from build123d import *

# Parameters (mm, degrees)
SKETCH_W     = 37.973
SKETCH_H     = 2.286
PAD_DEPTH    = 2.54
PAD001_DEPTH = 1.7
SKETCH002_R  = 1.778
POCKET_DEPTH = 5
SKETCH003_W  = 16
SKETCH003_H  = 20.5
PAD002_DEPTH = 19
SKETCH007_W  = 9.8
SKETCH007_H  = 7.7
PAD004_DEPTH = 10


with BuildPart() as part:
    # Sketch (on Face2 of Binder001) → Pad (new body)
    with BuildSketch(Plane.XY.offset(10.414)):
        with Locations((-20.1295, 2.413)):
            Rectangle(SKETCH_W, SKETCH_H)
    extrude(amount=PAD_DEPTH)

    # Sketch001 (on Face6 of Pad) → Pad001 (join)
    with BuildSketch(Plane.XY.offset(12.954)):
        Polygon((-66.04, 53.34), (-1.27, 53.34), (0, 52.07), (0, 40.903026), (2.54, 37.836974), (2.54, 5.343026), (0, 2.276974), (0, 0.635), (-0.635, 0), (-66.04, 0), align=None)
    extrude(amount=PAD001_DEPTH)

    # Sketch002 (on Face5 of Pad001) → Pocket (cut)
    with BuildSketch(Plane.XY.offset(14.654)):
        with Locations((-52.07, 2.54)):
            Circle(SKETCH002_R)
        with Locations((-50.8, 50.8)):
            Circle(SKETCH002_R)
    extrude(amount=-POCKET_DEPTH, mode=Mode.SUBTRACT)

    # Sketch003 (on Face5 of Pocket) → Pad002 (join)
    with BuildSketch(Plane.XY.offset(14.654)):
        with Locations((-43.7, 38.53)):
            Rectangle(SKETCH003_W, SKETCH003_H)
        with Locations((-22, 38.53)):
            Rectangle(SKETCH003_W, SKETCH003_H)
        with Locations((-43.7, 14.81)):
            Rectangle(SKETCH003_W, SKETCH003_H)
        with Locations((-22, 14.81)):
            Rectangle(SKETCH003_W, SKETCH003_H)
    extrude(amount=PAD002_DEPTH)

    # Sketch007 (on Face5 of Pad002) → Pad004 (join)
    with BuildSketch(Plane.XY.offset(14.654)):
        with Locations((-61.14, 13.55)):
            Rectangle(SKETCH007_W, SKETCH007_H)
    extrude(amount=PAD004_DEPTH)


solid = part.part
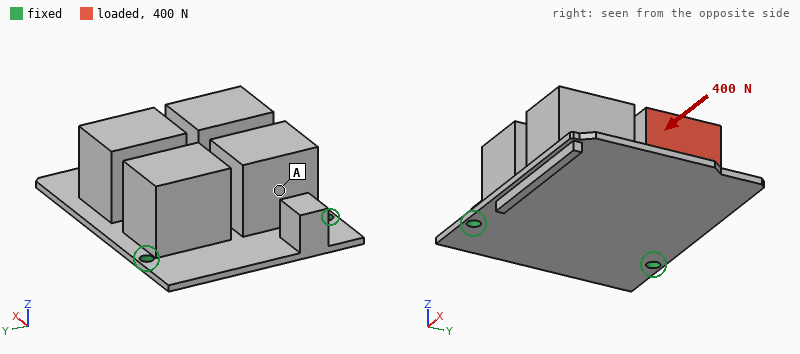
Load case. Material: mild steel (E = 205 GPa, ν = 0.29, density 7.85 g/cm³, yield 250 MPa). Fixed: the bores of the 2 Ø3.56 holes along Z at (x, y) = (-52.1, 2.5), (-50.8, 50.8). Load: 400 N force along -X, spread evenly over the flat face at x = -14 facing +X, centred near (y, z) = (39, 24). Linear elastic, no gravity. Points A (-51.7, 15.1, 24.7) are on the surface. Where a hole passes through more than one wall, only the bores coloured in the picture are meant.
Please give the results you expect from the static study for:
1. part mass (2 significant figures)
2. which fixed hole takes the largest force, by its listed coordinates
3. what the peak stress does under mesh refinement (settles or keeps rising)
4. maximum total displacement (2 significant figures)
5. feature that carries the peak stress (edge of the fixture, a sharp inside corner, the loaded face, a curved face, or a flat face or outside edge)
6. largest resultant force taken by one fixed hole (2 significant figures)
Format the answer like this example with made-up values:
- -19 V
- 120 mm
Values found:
- 250 g
- (-50.8, 50.8)
- keeps rising
- 0.33 mm
- edge of the fixture
- 300 N
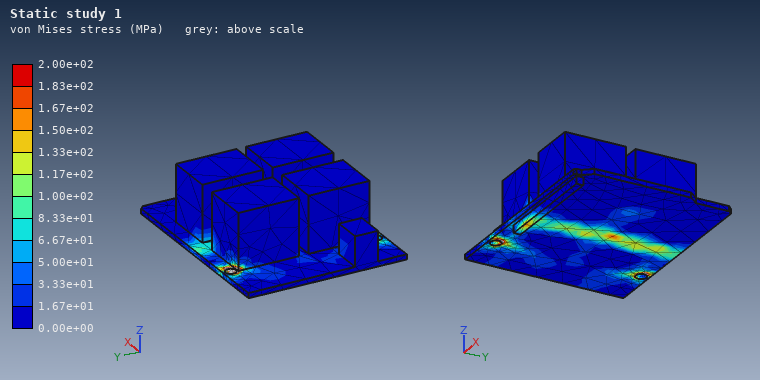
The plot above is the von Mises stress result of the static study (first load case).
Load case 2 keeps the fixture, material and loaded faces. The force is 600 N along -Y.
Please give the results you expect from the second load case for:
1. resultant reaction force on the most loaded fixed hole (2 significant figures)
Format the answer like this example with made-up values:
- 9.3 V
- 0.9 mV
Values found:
- 570 N
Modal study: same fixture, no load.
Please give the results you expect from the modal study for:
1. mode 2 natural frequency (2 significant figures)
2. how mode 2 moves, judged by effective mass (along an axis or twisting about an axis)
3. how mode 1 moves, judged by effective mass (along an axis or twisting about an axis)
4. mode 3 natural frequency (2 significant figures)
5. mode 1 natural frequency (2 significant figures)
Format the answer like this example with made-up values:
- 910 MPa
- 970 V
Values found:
- 1500 Hz
- along Z
- along Z
- 1900 Hz
- 420 Hz
